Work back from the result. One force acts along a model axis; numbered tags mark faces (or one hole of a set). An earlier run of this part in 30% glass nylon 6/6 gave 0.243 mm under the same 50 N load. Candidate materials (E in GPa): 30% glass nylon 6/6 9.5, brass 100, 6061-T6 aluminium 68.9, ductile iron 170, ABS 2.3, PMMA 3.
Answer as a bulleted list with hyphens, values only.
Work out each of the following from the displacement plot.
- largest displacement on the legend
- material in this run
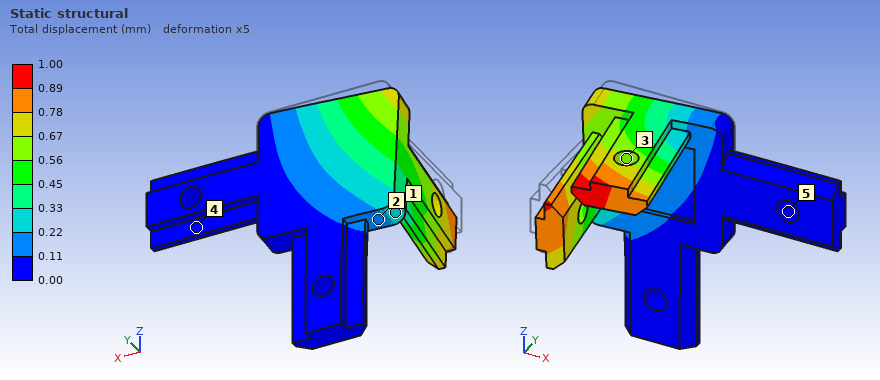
- 1.00 mm
- ABS
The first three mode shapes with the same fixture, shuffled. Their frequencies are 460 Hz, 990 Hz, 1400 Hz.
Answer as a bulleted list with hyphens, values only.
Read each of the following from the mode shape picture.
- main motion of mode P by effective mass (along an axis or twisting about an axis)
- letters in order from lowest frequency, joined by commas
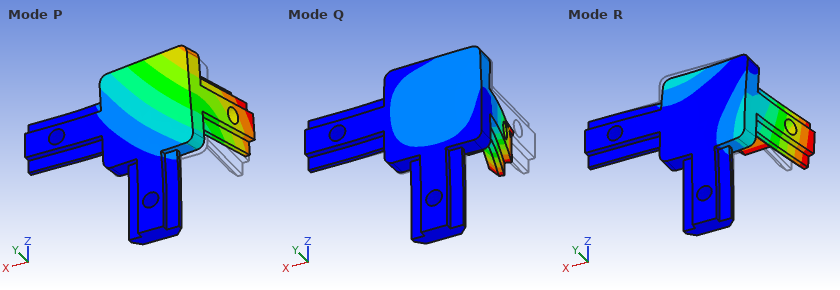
- along Y
- P, R, Q
